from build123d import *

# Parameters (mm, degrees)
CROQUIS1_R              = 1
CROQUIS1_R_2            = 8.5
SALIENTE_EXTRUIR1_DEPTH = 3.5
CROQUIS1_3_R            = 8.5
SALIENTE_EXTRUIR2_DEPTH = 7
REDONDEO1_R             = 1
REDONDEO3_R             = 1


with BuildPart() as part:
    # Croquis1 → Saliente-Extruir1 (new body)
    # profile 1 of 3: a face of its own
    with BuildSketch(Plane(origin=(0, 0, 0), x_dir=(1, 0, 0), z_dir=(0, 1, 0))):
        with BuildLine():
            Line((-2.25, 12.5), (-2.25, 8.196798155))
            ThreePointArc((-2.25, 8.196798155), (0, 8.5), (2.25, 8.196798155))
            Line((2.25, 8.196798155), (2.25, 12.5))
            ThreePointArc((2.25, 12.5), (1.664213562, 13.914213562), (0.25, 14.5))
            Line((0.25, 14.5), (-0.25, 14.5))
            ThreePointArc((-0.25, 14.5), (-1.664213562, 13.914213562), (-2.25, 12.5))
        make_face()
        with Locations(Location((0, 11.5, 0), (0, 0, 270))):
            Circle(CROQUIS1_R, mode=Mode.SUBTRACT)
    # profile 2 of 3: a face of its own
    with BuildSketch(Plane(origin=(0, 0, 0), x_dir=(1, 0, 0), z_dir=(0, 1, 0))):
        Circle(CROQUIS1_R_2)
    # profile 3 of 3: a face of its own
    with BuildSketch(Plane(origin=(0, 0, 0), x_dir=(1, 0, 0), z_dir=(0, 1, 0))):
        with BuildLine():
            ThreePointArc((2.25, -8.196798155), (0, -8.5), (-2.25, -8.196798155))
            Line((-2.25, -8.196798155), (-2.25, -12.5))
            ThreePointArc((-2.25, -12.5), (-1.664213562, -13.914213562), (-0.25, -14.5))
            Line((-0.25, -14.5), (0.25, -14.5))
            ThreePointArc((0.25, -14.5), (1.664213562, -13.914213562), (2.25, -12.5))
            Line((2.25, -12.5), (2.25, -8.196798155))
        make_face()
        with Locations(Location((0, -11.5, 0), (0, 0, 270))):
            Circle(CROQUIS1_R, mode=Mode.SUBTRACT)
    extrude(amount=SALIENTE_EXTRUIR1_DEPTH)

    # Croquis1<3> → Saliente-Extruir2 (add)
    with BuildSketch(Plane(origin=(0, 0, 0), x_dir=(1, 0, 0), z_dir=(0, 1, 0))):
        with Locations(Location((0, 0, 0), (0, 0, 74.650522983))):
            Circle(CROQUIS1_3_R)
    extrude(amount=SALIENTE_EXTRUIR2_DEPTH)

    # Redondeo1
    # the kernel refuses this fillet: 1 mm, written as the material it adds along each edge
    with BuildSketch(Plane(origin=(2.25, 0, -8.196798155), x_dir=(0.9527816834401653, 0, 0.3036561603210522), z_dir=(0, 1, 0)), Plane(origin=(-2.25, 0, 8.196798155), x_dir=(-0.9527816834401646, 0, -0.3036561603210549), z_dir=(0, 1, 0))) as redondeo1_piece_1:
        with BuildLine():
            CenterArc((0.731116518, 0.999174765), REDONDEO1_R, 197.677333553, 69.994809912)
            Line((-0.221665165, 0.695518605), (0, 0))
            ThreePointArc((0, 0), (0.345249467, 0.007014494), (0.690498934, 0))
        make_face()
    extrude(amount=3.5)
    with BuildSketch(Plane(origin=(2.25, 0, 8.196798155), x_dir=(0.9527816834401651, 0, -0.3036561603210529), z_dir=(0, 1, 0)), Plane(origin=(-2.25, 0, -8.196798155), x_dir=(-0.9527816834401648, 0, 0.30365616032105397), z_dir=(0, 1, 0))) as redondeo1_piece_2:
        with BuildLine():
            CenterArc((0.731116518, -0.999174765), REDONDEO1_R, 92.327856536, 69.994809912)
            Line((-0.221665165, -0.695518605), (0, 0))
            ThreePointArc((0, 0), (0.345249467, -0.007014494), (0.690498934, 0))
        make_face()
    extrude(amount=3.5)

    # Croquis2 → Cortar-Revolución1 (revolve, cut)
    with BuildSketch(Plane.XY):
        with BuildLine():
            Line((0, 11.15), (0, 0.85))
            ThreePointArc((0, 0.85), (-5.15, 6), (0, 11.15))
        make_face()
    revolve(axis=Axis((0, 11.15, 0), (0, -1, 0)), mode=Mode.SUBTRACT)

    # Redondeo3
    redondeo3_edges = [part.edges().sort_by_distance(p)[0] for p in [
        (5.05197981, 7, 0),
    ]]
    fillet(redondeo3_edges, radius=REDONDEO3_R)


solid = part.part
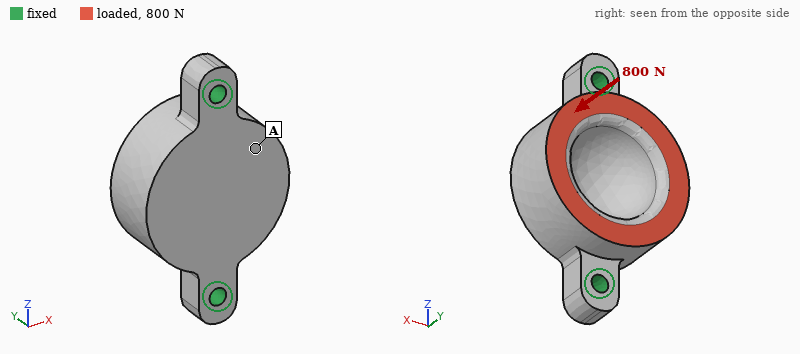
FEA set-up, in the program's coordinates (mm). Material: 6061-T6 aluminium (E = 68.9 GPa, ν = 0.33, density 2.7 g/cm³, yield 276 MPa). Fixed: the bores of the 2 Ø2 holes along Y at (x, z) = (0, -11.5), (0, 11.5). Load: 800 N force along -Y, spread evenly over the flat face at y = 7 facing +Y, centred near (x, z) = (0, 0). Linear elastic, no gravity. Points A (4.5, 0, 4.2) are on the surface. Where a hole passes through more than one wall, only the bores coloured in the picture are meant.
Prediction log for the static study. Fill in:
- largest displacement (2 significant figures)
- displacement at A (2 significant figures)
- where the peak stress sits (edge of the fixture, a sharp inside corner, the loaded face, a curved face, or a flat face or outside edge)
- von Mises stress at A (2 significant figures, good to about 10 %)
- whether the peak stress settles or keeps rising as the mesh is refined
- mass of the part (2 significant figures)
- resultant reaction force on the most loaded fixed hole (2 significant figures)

18 µm
12 µm
edge of the fixture
20 MPa
keeps rising
3.7 g
400 N
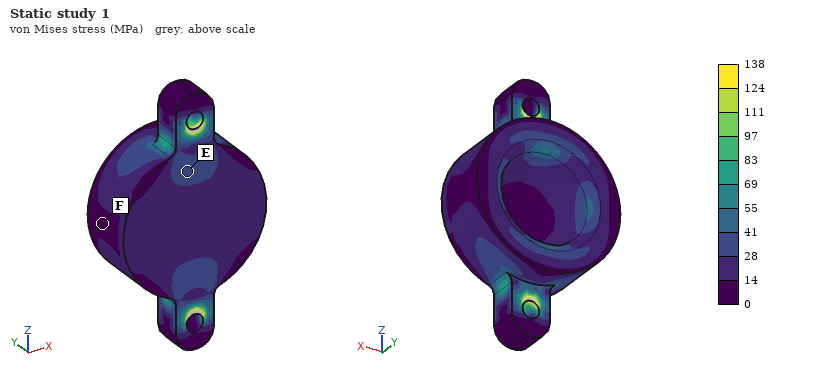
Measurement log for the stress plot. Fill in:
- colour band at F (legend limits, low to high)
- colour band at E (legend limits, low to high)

0 to 14 MPa
28 to 41 MPa
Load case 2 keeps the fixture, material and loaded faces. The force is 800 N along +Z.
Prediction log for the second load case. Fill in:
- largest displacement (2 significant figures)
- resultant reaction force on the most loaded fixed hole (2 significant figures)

6.2 µm
450 N
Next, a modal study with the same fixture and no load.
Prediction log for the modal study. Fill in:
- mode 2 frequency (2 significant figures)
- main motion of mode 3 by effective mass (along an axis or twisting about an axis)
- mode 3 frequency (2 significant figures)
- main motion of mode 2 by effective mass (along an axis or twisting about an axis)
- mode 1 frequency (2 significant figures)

22 kHz
along X
33 kHz
along Y
12 kHz
